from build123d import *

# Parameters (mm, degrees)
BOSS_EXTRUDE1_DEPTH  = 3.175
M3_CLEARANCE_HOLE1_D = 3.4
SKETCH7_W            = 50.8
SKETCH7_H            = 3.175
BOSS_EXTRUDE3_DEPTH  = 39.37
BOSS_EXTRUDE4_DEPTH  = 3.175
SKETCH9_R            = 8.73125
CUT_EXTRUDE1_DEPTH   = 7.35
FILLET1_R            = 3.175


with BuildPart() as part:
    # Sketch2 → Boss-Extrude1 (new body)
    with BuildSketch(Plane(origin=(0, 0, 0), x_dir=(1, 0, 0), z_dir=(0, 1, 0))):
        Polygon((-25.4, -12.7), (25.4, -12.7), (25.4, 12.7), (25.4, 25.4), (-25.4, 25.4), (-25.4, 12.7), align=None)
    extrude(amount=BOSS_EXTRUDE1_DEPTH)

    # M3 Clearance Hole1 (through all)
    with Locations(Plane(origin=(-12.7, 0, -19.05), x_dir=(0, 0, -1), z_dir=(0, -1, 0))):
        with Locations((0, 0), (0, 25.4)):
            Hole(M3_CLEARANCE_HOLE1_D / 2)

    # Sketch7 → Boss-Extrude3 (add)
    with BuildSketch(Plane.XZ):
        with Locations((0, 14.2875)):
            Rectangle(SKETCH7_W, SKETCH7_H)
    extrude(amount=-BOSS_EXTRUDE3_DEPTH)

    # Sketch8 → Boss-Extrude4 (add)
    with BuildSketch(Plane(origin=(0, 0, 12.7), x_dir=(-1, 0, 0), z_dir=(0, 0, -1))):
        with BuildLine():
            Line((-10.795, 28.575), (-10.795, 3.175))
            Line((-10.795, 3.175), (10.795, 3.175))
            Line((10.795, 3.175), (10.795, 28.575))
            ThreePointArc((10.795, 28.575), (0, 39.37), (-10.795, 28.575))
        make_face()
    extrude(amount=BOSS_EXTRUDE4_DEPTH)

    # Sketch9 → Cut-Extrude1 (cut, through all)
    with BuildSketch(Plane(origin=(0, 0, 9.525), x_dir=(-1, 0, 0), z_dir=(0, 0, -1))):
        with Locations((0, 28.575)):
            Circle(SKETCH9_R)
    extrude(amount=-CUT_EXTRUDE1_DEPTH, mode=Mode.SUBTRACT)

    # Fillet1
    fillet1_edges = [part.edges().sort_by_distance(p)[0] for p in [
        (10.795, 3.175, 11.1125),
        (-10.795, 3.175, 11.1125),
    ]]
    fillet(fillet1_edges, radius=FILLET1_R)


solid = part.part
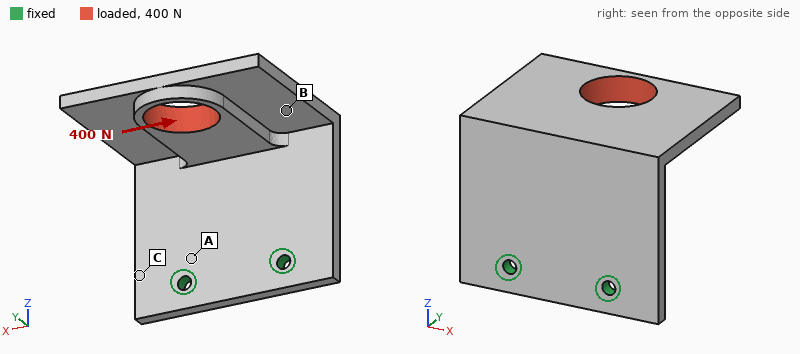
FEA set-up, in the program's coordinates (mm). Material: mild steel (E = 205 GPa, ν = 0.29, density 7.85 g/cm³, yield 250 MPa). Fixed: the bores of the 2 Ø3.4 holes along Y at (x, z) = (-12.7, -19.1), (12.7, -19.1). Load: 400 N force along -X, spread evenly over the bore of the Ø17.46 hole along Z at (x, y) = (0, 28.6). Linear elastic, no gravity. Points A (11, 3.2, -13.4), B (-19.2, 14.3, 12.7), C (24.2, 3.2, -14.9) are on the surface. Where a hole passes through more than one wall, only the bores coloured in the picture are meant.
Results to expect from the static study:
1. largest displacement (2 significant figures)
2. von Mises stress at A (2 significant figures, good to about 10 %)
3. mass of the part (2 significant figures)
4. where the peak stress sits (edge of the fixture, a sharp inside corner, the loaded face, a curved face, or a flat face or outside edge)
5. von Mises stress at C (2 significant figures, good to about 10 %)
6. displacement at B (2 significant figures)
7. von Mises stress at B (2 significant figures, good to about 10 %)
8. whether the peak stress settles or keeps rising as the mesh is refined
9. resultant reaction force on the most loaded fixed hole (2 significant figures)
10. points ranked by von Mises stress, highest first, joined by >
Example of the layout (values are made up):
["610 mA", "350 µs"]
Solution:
["0.19 mm", "79 MPa", "100 g", "edge of the fixture", "57 MPa", "0.097 mm", "16 MPa", "keeps rising", "600 N", "A > C > B"]
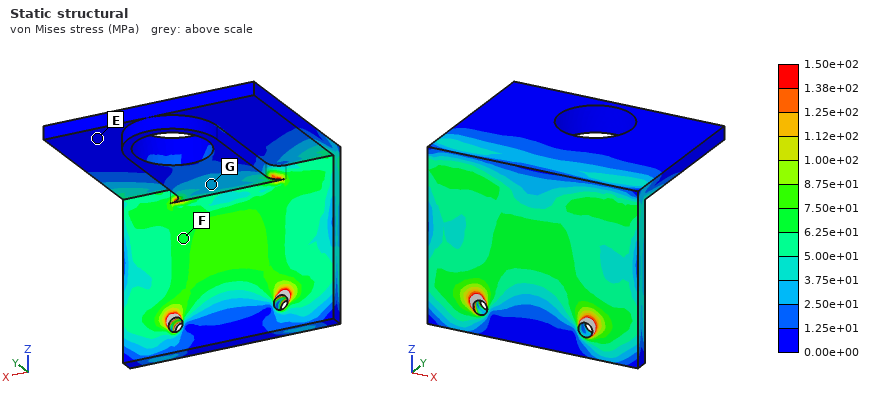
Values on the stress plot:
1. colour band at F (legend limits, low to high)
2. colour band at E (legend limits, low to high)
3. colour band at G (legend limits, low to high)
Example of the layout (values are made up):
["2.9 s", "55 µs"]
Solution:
["6.25e+01 to 7.50e+01 MPa", "0.00e+00 to 1.25e+01 MPa", "2.50e+01 to 3.75e+01 MPa"]
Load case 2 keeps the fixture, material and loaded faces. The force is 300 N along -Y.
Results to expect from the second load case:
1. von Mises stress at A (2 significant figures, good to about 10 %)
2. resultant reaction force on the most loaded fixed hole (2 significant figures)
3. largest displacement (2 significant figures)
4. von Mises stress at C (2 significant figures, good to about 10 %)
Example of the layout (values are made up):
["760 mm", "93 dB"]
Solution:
["99 MPa", "150 N", "0.26 mm", "68 MPa"]
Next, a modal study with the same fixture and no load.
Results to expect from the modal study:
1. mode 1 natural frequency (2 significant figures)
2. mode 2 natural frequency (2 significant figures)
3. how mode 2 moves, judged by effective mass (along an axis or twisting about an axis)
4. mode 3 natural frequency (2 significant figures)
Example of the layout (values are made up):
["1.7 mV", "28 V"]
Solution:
["700 Hz", "1300 Hz", "along X", "2400 Hz"]
